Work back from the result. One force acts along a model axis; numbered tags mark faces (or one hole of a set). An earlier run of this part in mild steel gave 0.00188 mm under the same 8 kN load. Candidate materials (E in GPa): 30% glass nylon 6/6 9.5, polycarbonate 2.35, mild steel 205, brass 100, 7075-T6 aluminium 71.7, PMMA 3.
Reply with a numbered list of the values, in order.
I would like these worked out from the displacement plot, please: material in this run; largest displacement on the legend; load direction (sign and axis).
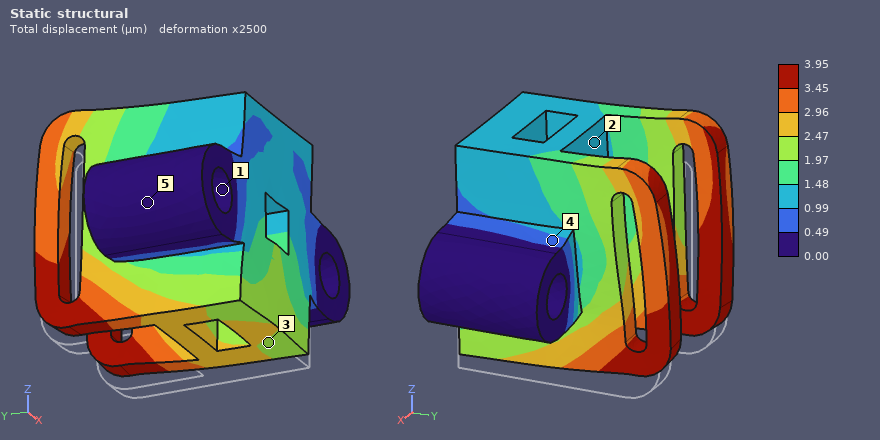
1. brass
2. 3.95 µm
3. +Z
